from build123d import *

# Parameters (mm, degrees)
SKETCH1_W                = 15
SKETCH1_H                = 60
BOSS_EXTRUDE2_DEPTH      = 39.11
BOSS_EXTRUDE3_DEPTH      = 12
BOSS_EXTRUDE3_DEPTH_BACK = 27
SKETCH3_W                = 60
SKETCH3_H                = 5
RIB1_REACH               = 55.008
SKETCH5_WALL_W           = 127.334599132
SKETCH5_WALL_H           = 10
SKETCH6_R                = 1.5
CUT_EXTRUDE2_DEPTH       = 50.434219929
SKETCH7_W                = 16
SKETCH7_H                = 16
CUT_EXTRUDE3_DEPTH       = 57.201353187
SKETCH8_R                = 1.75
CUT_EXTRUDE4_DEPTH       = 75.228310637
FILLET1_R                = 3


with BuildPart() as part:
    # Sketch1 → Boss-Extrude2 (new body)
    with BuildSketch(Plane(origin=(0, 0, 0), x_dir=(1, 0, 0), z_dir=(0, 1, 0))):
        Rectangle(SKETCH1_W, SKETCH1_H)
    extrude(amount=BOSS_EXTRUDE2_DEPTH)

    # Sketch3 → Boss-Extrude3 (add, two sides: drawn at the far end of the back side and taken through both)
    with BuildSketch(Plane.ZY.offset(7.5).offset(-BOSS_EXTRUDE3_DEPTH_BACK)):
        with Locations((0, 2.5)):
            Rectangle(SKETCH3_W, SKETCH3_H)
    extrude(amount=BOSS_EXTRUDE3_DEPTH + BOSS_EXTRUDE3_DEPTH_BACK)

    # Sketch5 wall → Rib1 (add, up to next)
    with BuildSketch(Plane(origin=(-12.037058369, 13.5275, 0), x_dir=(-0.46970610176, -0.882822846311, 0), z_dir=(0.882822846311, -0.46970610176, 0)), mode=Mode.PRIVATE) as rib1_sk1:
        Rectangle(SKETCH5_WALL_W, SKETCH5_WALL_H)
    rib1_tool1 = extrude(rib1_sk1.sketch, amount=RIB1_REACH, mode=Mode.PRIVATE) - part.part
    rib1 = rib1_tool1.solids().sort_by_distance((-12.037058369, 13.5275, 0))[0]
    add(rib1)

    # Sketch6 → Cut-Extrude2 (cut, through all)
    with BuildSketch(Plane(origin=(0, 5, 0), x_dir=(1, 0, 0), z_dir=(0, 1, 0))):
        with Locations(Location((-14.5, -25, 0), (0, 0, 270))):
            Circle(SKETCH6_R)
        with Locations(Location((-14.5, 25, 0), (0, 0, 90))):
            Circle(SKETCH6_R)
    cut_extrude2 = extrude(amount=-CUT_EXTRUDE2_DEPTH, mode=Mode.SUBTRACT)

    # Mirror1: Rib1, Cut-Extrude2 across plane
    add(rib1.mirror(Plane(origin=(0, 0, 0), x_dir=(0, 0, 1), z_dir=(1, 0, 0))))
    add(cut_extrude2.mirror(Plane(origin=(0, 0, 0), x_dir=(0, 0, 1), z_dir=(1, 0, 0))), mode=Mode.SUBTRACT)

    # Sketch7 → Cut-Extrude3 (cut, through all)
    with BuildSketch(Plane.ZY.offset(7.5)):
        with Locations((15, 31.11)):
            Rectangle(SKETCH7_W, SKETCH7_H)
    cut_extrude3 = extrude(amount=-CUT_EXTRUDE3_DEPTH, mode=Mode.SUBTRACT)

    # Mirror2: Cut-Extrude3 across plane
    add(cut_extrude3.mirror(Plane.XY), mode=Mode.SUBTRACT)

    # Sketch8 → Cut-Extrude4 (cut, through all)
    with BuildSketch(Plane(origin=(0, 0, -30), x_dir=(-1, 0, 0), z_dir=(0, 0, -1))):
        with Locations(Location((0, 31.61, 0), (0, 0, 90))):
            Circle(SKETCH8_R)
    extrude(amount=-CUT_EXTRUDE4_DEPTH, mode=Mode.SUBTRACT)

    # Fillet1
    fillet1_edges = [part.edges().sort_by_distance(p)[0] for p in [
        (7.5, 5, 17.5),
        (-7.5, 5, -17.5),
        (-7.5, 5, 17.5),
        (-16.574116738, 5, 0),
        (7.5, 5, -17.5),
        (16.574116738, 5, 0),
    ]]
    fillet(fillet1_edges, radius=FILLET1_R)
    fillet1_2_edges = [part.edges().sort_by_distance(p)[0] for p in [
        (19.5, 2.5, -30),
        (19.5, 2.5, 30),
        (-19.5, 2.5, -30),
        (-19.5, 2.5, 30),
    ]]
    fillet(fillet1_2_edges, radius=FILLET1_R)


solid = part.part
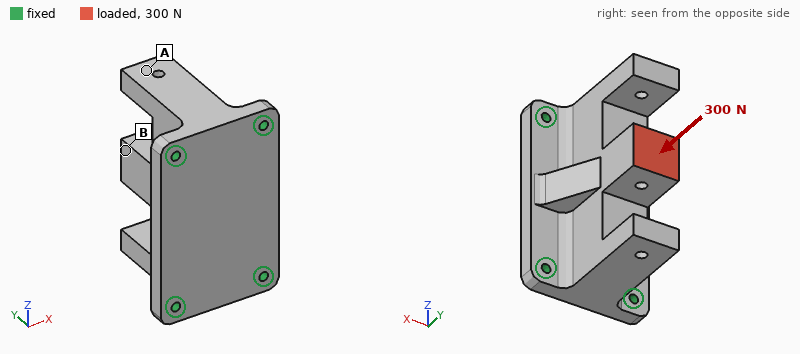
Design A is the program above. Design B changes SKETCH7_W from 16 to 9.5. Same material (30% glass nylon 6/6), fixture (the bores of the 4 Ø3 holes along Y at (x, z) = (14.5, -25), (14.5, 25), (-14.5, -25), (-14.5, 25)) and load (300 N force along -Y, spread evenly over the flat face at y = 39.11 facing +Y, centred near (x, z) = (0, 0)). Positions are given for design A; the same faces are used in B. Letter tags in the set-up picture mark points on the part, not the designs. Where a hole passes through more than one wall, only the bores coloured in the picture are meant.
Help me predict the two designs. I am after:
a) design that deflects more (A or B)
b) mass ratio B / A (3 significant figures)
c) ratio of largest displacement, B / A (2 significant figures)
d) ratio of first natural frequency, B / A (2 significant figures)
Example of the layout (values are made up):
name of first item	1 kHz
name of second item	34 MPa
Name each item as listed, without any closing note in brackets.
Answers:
design that deflects more	A
mass ratio B / A	1.08
ratio of largest displacement, B / A	0.87
ratio of first natural frequency, B / A	0.89
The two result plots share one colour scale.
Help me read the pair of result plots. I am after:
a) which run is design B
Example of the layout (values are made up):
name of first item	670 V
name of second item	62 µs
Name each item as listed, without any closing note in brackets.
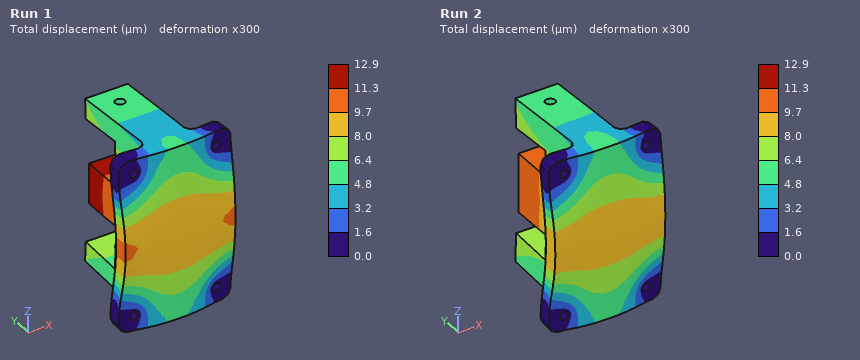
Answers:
which run is design B	Run 2
